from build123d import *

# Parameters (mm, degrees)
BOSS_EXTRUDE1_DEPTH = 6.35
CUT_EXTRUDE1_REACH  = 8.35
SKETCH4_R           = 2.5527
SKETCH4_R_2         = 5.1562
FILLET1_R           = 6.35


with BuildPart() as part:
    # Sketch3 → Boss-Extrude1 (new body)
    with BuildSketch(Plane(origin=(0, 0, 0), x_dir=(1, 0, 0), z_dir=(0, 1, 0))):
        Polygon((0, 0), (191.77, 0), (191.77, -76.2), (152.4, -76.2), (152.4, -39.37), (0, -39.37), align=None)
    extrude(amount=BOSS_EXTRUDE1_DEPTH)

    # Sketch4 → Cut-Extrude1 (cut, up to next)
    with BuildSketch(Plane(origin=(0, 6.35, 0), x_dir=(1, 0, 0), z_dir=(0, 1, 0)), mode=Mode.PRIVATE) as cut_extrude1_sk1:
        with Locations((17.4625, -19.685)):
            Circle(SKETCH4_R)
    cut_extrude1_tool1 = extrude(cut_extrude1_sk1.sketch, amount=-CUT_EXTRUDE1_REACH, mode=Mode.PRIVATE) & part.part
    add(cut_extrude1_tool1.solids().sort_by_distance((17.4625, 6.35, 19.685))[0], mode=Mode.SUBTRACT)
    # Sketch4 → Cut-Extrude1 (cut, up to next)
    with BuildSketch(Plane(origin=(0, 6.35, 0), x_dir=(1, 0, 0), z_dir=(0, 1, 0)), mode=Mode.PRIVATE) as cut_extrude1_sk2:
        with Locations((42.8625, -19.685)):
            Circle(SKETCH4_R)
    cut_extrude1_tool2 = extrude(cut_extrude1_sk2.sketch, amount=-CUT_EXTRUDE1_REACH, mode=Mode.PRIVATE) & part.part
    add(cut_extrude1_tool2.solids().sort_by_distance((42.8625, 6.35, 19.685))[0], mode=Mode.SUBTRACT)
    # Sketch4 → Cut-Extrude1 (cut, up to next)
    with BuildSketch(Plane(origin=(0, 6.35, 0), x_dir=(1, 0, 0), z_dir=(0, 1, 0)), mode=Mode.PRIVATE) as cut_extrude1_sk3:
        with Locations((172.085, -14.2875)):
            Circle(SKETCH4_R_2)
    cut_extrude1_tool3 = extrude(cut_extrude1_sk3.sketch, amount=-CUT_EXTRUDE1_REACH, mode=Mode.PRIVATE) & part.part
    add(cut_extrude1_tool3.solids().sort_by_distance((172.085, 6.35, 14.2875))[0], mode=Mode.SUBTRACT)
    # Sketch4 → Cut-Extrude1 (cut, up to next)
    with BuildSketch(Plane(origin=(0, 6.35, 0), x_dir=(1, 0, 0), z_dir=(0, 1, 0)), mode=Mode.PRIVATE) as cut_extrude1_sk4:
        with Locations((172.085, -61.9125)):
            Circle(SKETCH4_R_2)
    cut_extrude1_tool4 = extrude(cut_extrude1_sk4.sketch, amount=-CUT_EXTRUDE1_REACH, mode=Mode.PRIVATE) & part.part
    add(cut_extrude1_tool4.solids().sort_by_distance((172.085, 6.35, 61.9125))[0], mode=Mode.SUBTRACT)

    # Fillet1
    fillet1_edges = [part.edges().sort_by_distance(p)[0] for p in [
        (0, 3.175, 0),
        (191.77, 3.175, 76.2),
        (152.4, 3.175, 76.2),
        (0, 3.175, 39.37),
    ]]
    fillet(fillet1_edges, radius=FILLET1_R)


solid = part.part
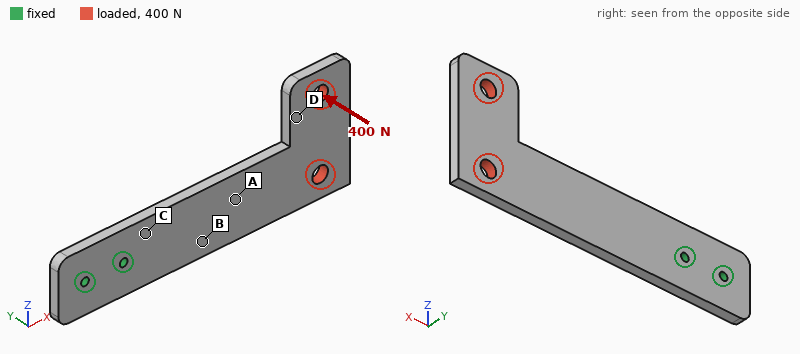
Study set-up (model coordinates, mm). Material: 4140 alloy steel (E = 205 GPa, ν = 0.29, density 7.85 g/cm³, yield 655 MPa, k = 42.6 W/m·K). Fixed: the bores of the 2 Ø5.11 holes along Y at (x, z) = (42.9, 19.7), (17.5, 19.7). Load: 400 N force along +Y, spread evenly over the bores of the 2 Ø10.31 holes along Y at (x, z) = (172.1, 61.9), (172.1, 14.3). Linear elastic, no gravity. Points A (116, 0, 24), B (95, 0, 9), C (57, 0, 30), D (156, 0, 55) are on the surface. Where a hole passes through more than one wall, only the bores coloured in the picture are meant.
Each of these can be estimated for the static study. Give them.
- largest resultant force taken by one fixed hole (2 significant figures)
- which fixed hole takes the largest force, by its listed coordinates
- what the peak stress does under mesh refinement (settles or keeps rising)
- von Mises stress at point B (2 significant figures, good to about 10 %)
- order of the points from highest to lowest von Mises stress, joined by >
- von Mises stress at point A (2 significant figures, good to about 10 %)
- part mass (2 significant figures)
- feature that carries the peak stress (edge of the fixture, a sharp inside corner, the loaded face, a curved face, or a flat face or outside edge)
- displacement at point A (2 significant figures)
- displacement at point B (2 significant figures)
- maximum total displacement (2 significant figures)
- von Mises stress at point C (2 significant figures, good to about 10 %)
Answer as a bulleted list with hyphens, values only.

- 1.2 kN
- (42.9, 19.7)
- keeps rising
- 120 MPa
- C > B > A > D
- 88 MPa
- 440 g
- edge of the fixture
- 0.70 mm
- 0.35 mm
- 2.3 mm
- 170 MPa
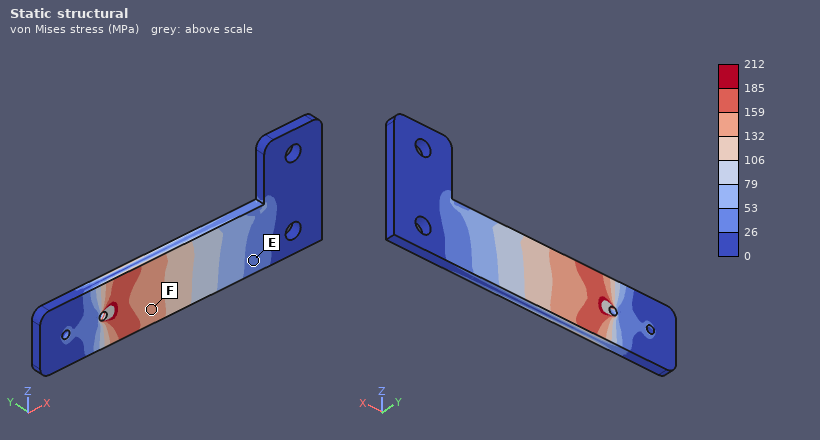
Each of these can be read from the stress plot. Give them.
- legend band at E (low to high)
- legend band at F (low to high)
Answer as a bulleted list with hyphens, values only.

- 26 to 53 MPa
- 132 to 159 MPa
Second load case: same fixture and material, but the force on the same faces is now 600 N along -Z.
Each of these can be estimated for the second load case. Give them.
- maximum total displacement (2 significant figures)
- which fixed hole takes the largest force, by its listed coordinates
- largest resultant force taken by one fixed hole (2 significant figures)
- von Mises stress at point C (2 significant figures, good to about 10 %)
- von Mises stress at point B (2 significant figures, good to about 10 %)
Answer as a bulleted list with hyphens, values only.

- 0.14 mm
- (42.9, 19.7)
- 3.1 kN
- 23 MPa
- 16 MPa
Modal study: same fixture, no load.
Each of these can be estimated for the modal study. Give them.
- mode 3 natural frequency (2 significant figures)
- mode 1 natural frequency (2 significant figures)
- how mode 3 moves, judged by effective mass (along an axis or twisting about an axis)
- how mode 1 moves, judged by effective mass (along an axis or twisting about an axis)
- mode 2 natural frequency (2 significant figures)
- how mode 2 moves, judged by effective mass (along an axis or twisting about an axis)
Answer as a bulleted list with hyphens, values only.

- 870 Hz
- 180 Hz
- along Z
- along Y
- 750 Hz
- twisting about X
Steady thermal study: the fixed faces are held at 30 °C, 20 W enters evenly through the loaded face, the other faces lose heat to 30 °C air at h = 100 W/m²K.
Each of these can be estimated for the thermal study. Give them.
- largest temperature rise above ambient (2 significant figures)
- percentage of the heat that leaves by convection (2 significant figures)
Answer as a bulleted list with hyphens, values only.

- 32 K
- 98 %
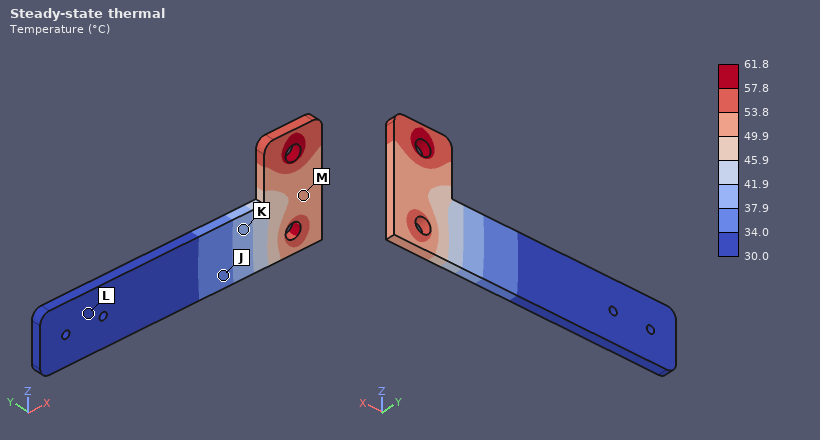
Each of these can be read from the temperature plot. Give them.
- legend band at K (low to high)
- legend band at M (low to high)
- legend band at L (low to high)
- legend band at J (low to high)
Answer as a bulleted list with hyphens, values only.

- 37.9 to 41.9 °C
- 49.9 to 53.8 °C
- 30.0 to 34.0 °C
- 34.0 to 37.9 °C
